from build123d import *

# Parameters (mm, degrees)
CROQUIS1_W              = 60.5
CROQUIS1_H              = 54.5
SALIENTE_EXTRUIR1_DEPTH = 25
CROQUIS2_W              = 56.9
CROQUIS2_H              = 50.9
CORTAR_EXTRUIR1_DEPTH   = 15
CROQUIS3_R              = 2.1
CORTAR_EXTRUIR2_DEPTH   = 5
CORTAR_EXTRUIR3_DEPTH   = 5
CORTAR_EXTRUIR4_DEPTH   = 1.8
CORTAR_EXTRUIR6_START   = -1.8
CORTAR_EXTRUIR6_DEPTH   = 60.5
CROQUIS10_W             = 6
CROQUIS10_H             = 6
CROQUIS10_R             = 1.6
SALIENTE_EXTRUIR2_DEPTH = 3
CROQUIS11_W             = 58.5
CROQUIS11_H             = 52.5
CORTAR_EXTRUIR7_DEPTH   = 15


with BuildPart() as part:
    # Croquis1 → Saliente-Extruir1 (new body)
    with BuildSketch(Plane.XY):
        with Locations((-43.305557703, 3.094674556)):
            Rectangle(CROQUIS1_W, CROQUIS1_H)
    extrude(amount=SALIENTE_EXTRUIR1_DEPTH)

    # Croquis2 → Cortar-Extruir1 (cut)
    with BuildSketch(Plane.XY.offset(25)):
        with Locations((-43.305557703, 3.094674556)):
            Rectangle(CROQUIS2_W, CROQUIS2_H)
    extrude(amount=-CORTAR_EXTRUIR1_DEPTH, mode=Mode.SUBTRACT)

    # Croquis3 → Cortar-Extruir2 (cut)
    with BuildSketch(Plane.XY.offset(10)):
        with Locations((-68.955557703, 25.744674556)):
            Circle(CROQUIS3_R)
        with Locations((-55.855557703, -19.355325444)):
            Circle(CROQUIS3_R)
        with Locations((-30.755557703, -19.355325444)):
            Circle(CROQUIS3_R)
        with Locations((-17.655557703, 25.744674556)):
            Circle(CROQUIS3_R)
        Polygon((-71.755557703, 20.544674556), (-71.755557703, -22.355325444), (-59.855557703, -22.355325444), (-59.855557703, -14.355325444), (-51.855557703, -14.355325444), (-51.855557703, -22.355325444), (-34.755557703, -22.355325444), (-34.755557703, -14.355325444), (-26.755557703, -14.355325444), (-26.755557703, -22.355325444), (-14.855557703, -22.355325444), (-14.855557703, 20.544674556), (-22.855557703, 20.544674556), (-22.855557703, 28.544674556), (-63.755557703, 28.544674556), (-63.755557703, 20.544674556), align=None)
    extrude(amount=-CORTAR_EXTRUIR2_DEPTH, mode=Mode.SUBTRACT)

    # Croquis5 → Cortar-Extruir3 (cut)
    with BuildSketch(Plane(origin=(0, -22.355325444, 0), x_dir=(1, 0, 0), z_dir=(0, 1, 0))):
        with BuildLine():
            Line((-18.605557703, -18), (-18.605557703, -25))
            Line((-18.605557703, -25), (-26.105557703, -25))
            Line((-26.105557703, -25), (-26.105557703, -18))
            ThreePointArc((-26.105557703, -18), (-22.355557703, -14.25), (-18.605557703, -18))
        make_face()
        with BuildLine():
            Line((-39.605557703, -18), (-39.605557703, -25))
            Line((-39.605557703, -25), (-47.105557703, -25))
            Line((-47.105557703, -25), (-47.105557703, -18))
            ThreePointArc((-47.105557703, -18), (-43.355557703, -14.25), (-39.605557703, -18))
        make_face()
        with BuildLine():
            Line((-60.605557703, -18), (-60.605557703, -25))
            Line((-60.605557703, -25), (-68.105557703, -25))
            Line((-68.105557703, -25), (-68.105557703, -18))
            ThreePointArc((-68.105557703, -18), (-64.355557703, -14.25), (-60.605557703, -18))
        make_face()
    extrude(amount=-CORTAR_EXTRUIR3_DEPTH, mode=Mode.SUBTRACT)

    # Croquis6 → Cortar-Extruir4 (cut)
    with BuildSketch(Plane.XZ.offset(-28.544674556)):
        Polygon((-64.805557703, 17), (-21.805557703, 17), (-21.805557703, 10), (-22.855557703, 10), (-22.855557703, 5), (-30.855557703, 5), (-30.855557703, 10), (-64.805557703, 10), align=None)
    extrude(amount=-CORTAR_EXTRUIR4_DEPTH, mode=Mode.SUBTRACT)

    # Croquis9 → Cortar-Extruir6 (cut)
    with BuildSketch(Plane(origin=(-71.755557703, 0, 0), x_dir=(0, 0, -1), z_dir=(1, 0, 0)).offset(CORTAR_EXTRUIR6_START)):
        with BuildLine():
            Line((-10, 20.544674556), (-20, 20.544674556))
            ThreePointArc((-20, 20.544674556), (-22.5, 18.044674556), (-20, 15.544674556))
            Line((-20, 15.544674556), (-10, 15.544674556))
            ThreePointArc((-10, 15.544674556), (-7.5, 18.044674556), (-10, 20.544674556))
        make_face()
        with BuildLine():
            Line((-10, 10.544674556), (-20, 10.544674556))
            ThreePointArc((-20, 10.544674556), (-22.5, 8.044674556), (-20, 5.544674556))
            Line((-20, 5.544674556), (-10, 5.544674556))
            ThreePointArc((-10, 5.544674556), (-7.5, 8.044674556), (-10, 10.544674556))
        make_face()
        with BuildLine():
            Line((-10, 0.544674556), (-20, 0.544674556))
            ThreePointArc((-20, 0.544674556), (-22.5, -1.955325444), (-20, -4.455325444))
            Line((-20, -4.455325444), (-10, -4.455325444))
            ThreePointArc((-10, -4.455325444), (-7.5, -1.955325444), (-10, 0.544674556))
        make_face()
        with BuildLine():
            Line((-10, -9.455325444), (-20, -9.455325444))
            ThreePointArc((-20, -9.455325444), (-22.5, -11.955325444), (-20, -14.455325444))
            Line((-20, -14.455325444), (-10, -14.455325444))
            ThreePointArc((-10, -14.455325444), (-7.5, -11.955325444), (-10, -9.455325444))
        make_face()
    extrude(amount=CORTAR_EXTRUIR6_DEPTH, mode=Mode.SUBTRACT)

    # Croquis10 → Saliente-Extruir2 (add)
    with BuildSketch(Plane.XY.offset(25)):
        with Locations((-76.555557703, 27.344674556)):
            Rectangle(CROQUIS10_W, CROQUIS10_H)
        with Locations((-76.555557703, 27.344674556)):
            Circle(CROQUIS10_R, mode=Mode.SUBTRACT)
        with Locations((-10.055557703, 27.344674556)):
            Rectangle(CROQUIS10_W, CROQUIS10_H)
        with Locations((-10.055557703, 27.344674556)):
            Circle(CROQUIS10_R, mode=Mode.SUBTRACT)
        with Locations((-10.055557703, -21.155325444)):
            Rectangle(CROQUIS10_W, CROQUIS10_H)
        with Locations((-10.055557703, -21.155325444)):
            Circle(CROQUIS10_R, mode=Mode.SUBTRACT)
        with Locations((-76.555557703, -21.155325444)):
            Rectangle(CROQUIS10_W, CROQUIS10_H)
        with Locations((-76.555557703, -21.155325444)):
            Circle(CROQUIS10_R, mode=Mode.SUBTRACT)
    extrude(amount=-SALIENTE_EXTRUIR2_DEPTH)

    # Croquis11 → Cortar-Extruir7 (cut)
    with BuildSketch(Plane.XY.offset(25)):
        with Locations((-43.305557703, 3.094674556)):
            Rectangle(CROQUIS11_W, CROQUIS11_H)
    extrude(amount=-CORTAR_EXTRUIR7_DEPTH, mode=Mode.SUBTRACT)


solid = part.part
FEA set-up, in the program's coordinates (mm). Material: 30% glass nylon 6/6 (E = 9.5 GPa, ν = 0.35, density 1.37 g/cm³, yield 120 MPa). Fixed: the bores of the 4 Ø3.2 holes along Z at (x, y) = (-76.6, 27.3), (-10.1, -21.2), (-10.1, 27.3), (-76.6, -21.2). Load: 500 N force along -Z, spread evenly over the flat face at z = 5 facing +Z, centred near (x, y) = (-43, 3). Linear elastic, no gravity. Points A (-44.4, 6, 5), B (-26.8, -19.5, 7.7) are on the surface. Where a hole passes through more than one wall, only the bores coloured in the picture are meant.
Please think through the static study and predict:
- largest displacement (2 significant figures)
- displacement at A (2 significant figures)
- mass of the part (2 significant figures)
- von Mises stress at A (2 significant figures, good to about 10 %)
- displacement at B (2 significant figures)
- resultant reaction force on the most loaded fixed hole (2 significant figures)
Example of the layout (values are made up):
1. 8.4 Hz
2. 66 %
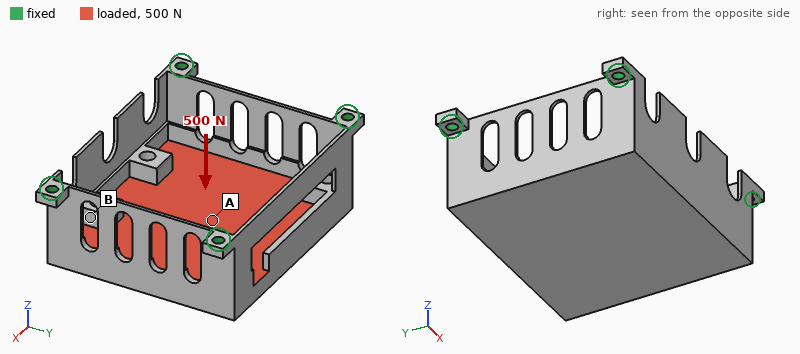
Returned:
1. 0.13 mm
2. 0.13 mm
3. 30 g
4. 6.9 MPa
5. 0.058 mm
6. 130 N
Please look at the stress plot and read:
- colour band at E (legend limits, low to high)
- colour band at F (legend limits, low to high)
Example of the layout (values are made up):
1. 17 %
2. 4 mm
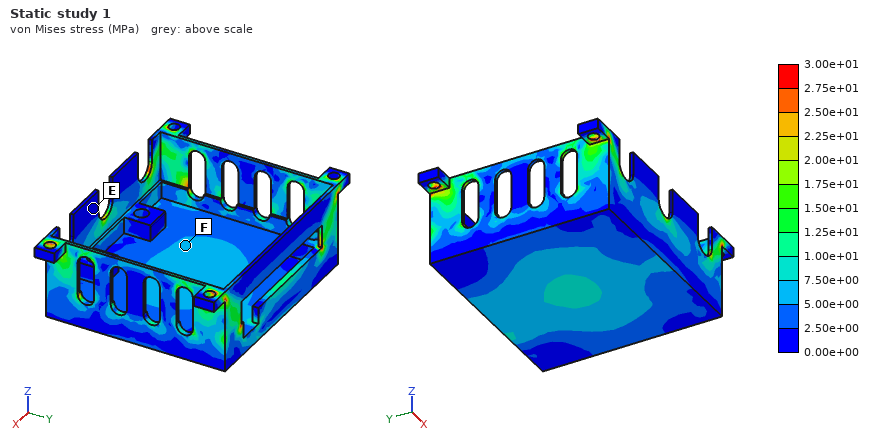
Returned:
1. 0.00e+00 to 2.50e+00 MPa
2. 5.00e+00 to 7.50e+00 MPa
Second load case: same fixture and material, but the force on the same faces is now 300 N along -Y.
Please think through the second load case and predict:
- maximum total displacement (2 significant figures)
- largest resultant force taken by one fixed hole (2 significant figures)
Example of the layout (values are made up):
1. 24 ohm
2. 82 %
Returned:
1. 88 µm
2. 92 N
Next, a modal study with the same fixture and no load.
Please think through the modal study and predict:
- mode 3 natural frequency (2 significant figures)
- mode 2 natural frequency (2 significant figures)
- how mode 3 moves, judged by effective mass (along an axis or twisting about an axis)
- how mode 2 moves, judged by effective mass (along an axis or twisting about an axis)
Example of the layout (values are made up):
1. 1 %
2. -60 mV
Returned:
1. 1800 Hz
2. 1500 Hz
3. along Y
4. along X
